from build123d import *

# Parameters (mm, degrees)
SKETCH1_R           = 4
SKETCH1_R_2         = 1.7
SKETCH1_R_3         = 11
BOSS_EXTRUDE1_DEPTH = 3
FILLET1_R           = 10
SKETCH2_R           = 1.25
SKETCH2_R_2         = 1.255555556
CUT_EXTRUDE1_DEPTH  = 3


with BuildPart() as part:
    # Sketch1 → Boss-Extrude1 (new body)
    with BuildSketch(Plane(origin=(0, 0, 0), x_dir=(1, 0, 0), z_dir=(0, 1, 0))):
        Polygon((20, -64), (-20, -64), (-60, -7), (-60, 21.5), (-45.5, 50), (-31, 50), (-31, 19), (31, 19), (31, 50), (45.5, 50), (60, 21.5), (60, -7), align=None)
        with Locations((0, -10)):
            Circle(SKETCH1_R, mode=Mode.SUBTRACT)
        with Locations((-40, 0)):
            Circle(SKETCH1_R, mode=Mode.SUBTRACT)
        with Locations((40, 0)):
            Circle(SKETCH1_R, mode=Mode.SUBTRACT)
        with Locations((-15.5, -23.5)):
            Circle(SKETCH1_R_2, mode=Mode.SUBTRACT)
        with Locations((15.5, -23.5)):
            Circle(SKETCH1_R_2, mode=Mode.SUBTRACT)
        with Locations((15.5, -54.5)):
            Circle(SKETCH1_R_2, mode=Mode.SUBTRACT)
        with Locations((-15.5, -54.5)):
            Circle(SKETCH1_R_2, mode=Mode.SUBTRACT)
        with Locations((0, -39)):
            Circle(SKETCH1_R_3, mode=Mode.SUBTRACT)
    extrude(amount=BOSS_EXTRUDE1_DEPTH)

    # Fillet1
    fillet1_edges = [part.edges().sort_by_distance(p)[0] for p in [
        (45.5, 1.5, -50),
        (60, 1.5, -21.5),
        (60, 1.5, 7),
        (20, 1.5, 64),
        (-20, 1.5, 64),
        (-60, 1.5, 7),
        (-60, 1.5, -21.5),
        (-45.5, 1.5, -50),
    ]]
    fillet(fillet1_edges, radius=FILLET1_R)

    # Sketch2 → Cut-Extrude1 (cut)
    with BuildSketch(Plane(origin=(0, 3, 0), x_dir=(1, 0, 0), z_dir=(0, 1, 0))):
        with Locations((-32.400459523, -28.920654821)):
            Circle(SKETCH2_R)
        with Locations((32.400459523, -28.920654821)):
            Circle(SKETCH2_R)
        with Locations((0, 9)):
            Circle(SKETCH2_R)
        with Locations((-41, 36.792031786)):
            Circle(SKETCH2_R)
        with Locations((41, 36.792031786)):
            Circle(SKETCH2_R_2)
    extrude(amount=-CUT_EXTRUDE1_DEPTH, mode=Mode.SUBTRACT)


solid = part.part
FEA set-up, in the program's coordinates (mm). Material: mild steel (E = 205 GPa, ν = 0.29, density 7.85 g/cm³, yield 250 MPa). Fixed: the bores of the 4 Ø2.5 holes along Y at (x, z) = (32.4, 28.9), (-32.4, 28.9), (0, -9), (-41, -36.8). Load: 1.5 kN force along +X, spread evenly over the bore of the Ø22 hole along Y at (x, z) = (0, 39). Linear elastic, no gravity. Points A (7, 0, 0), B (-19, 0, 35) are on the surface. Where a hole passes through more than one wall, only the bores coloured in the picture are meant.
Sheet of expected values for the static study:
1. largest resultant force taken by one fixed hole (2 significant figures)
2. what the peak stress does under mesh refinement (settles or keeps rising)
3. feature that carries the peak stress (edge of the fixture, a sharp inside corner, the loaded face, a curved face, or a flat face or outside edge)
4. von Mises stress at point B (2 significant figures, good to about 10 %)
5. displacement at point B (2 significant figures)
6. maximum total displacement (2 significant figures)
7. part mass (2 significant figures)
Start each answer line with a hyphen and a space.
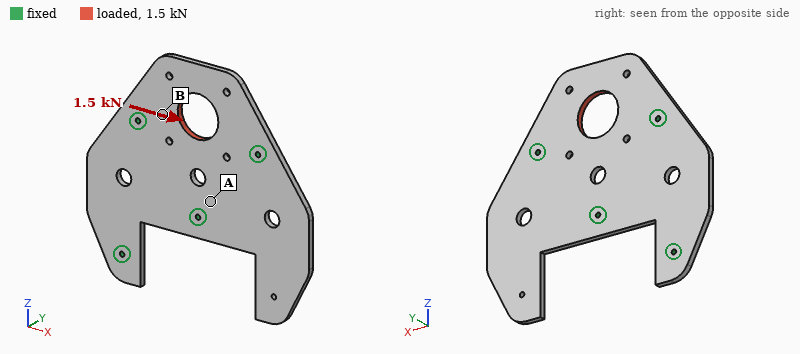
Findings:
- 750 N
- keeps rising
- edge of the fixture
- 12 MPa
- 1.4 µm
- 3.3 µm
- 200 g
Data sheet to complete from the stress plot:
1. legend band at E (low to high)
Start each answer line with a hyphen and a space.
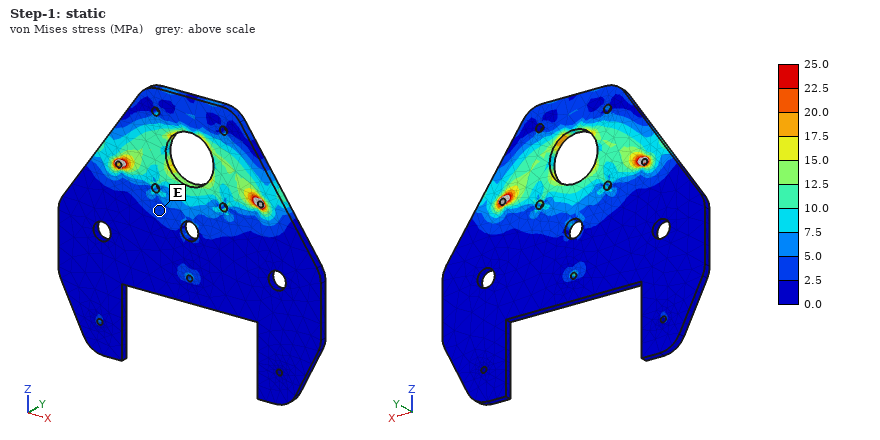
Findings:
- 2.5 to 5.0 MPa
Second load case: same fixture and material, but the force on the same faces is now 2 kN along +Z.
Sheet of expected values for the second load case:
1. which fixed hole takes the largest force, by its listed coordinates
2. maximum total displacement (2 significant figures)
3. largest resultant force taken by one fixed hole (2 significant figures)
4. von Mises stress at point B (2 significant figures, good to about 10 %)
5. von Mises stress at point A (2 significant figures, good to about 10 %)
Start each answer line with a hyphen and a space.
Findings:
- (32.4, 28.9)
- 3.7 µm
- 740 N
- 11 MPa
- 9.6 MPa
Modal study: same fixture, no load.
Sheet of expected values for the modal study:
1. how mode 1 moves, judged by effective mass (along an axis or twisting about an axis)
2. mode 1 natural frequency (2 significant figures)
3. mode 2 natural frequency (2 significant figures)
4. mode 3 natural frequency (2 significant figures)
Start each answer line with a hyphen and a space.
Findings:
- along Y
- 720 Hz
- 1600 Hz
- 2100 Hz
